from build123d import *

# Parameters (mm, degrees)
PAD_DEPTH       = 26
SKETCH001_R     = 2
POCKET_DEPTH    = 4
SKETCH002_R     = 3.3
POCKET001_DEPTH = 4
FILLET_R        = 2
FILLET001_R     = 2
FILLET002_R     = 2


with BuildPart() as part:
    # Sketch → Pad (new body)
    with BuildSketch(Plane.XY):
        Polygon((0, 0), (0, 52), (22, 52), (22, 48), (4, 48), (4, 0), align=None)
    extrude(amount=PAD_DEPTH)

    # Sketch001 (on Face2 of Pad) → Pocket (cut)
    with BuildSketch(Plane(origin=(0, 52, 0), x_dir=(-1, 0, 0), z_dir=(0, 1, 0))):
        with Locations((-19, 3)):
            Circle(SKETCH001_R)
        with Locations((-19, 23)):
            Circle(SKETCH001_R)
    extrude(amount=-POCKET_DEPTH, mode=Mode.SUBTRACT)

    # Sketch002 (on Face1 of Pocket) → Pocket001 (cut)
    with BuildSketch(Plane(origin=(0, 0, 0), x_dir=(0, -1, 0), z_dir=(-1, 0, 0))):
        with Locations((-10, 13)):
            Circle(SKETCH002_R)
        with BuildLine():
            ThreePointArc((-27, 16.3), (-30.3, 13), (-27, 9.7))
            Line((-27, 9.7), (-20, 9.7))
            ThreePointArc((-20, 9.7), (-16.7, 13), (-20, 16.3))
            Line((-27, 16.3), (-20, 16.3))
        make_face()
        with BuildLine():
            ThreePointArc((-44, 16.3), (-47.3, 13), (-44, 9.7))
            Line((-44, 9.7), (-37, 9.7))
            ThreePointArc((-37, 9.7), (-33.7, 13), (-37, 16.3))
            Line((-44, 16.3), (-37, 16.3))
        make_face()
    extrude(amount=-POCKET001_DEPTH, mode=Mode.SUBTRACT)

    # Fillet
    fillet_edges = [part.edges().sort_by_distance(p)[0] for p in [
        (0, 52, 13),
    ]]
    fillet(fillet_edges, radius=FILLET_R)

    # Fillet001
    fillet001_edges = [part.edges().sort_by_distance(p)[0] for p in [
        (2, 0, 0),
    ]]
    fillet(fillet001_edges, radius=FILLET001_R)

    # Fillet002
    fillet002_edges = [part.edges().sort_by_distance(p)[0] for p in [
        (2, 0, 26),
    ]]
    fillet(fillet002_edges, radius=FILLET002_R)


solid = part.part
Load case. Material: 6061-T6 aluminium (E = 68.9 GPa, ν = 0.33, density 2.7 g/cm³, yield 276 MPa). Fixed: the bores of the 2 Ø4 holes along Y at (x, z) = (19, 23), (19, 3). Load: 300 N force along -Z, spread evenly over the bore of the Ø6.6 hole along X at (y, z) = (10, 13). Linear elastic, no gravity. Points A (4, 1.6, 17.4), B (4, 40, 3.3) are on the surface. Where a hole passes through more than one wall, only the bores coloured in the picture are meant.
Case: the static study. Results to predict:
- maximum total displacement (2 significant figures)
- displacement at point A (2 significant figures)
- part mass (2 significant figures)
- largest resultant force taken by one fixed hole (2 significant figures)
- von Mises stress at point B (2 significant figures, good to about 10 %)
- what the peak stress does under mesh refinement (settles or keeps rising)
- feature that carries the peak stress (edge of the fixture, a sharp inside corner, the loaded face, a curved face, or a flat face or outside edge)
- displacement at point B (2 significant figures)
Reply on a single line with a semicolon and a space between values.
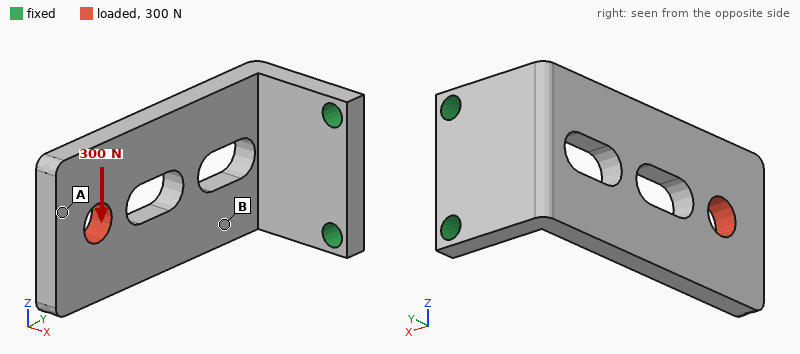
0.40 mm; 0.38 mm; 17 g; 650 N; 46 MPa; keeps rising; edge of the fixture; 0.11 mm
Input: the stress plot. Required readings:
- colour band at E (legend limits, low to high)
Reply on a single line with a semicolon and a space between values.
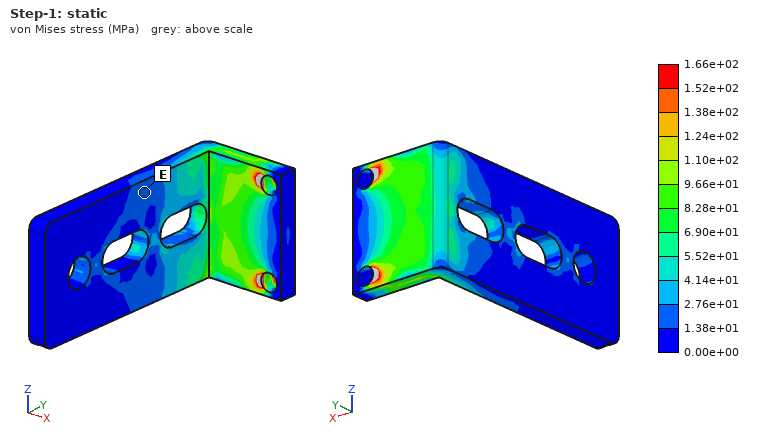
1.38e+01 to 2.76e+01 MPa
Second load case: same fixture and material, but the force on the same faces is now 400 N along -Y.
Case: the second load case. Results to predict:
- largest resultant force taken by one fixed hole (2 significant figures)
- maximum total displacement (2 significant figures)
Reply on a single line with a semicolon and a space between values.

200 N; 0.31 mm
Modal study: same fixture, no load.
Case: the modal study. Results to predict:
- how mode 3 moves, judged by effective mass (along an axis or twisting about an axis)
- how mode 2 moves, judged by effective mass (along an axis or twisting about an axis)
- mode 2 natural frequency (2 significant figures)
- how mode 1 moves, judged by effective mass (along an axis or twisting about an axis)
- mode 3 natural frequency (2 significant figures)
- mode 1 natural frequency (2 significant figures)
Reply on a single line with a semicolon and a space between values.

along Y; along Z; 1900 Hz; along X; 4000 Hz; 860 Hz
